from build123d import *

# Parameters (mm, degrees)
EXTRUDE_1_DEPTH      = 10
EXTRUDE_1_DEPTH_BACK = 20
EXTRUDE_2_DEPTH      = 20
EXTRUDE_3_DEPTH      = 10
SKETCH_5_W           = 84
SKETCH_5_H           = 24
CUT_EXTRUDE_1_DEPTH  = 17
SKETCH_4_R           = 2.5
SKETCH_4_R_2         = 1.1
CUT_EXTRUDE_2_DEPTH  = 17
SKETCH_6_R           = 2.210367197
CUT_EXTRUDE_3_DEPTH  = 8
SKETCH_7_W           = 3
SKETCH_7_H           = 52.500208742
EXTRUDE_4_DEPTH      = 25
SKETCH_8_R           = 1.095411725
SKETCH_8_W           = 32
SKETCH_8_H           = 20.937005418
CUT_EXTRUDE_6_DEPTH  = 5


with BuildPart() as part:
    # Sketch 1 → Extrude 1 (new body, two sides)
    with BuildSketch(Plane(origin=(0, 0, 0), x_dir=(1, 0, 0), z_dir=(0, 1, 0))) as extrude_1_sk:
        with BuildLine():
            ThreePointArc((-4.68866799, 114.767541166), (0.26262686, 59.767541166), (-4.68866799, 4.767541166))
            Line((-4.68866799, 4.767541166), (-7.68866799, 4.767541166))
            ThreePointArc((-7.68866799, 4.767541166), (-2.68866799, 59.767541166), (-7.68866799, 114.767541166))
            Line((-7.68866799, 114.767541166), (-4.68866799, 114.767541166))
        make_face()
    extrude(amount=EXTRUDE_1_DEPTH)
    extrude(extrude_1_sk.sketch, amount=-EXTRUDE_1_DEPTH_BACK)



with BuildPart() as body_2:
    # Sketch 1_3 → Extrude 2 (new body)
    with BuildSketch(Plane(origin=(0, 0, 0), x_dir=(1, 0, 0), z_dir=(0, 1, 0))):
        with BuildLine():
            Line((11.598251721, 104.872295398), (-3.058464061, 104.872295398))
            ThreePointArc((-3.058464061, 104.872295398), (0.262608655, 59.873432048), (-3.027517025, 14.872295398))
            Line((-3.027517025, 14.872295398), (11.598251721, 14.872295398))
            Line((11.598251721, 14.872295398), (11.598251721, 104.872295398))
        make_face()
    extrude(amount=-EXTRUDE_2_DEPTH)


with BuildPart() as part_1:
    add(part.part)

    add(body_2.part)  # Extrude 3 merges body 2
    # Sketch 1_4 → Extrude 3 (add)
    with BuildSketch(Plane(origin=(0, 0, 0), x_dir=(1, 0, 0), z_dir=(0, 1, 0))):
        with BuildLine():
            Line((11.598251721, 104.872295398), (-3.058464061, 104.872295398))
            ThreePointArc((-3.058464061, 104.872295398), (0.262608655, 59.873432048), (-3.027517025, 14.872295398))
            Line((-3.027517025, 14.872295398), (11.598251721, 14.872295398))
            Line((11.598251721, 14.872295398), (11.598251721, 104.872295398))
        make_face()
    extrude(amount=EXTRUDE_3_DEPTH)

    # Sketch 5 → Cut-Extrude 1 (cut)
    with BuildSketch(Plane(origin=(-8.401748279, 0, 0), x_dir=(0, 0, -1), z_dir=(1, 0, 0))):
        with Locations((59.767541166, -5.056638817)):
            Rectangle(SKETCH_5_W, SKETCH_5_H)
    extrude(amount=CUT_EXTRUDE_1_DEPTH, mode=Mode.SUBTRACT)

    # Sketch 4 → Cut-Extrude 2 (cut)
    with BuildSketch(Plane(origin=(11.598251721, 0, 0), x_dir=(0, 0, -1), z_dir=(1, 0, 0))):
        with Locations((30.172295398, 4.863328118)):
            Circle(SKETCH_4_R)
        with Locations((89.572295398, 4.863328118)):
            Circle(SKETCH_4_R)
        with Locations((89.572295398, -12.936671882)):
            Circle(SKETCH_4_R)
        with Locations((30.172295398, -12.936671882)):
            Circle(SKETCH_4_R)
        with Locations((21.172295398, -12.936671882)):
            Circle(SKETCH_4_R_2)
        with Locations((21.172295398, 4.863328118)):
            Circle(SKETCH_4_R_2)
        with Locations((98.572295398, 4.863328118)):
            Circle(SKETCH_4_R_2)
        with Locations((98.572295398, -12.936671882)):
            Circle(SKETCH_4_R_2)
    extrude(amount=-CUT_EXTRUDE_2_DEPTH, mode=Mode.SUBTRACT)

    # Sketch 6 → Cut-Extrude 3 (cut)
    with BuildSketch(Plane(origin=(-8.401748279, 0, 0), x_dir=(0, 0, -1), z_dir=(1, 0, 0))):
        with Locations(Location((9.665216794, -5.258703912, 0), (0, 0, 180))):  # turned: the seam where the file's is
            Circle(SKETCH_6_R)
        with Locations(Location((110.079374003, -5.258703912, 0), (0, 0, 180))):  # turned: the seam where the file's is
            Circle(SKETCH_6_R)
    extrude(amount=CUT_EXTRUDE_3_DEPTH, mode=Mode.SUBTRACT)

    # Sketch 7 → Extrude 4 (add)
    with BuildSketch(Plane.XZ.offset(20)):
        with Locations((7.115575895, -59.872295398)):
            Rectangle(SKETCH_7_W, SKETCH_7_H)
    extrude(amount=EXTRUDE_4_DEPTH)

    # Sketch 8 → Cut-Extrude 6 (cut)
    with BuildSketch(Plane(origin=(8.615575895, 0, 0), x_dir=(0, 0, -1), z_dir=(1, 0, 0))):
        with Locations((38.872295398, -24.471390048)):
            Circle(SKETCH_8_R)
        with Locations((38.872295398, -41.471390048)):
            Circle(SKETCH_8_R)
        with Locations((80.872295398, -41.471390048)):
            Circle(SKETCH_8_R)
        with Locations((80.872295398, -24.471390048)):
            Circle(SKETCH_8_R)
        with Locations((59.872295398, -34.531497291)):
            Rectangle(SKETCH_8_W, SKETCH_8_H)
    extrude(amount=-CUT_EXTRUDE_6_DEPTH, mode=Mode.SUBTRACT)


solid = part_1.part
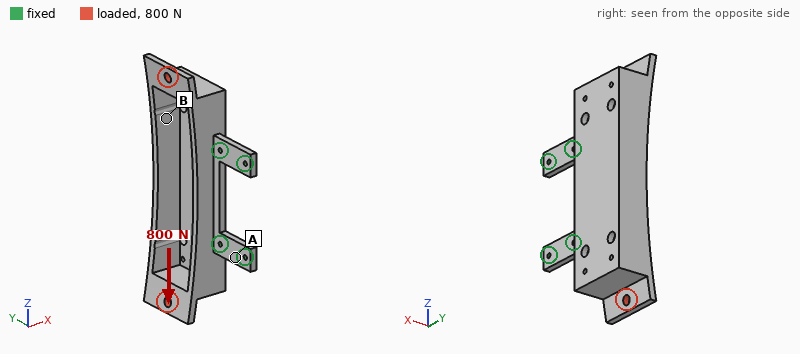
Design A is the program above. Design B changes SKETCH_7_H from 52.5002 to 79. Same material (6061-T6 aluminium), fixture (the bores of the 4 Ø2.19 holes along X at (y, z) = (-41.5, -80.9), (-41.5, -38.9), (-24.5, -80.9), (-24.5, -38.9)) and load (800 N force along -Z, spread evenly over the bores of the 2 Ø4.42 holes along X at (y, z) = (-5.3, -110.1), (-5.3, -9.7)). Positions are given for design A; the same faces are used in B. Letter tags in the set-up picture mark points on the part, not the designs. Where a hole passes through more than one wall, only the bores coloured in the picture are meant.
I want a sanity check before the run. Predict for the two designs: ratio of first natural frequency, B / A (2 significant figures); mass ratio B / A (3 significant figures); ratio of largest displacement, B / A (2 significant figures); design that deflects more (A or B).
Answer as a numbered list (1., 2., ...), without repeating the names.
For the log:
1. 1.3
2. 1.10
3. 0.84
4. A
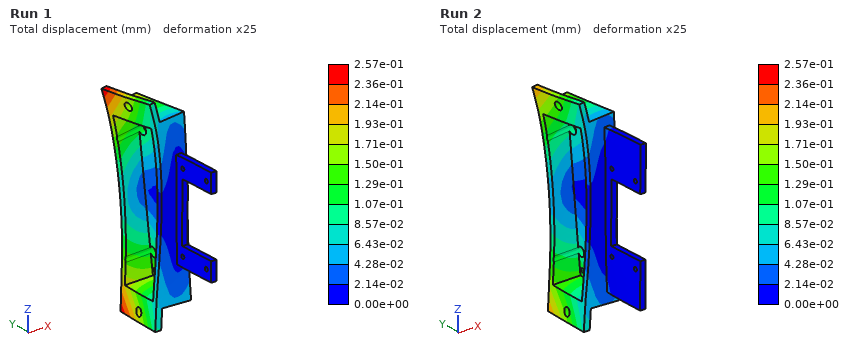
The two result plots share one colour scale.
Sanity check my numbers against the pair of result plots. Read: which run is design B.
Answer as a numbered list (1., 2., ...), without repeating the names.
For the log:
1. Run 2
